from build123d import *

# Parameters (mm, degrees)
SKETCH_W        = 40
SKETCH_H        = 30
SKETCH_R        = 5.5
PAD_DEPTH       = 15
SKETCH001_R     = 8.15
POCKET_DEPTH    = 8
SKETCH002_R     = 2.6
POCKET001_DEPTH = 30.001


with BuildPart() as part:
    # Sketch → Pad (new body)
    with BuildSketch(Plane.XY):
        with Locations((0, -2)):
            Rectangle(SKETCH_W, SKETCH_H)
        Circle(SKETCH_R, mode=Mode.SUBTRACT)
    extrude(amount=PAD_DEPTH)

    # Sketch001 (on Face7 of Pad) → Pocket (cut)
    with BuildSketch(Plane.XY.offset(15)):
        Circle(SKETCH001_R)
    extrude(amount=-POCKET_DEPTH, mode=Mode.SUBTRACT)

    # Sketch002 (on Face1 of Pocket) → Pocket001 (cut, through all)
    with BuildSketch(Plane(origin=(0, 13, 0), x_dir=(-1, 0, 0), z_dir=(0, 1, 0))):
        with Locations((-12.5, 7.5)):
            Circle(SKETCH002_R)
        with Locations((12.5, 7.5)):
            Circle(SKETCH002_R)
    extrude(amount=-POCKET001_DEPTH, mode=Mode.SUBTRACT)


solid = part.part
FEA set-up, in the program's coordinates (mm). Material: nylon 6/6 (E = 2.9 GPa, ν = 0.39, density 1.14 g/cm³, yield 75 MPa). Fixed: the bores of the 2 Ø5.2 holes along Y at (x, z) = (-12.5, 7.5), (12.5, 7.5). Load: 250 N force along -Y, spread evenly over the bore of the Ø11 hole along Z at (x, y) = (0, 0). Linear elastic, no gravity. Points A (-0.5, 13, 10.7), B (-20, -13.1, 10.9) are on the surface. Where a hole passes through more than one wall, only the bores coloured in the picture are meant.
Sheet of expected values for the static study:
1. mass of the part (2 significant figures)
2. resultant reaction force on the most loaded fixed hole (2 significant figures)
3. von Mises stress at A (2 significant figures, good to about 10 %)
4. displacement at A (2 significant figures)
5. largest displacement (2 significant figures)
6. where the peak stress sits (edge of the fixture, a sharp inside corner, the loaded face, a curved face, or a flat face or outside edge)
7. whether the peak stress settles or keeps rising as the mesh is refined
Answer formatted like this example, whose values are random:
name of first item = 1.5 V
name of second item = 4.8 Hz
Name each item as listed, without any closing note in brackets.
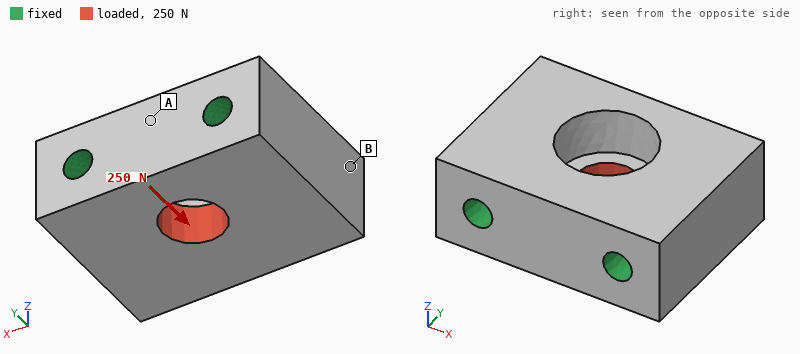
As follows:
mass of the part = 16 g
resultant reaction force on the most loaded fixed hole = 130 N
von Mises stress at A = 0.40 MPa
displacement at A = 2.3 µm
largest displacement = 8.1 µm
where the peak stress sits = edge of the fixture
whether the peak stress settles or keeps rising as the mesh is refined = keeps rising
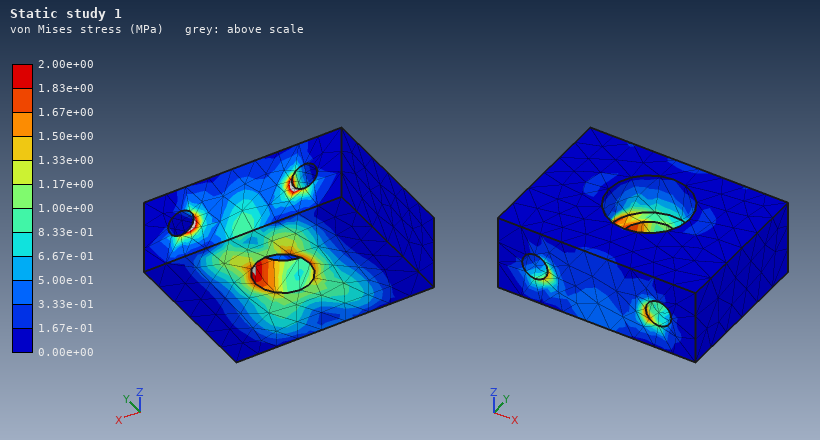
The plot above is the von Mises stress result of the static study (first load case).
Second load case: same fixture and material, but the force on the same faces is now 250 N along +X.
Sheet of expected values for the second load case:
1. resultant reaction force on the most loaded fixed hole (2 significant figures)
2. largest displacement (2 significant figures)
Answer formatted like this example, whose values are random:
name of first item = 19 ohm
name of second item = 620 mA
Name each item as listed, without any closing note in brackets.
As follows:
resultant reaction force on the most loaded fixed hole = 130 N
largest displacement = 4.4 µm
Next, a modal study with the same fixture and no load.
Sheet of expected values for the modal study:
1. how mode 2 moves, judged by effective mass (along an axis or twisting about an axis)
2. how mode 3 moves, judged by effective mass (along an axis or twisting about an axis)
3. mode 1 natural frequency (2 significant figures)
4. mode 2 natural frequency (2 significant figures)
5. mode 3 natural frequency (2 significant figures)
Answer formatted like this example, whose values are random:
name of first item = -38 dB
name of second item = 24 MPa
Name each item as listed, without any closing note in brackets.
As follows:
how mode 2 moves, judged by effective mass = twisting about X
how mode 3 moves, judged by effective mass = along Y
mode 1 natural frequency = 16 kHz
mode 2 natural frequency = 18 kHz
mode 3 natural frequency = 20 kHz
